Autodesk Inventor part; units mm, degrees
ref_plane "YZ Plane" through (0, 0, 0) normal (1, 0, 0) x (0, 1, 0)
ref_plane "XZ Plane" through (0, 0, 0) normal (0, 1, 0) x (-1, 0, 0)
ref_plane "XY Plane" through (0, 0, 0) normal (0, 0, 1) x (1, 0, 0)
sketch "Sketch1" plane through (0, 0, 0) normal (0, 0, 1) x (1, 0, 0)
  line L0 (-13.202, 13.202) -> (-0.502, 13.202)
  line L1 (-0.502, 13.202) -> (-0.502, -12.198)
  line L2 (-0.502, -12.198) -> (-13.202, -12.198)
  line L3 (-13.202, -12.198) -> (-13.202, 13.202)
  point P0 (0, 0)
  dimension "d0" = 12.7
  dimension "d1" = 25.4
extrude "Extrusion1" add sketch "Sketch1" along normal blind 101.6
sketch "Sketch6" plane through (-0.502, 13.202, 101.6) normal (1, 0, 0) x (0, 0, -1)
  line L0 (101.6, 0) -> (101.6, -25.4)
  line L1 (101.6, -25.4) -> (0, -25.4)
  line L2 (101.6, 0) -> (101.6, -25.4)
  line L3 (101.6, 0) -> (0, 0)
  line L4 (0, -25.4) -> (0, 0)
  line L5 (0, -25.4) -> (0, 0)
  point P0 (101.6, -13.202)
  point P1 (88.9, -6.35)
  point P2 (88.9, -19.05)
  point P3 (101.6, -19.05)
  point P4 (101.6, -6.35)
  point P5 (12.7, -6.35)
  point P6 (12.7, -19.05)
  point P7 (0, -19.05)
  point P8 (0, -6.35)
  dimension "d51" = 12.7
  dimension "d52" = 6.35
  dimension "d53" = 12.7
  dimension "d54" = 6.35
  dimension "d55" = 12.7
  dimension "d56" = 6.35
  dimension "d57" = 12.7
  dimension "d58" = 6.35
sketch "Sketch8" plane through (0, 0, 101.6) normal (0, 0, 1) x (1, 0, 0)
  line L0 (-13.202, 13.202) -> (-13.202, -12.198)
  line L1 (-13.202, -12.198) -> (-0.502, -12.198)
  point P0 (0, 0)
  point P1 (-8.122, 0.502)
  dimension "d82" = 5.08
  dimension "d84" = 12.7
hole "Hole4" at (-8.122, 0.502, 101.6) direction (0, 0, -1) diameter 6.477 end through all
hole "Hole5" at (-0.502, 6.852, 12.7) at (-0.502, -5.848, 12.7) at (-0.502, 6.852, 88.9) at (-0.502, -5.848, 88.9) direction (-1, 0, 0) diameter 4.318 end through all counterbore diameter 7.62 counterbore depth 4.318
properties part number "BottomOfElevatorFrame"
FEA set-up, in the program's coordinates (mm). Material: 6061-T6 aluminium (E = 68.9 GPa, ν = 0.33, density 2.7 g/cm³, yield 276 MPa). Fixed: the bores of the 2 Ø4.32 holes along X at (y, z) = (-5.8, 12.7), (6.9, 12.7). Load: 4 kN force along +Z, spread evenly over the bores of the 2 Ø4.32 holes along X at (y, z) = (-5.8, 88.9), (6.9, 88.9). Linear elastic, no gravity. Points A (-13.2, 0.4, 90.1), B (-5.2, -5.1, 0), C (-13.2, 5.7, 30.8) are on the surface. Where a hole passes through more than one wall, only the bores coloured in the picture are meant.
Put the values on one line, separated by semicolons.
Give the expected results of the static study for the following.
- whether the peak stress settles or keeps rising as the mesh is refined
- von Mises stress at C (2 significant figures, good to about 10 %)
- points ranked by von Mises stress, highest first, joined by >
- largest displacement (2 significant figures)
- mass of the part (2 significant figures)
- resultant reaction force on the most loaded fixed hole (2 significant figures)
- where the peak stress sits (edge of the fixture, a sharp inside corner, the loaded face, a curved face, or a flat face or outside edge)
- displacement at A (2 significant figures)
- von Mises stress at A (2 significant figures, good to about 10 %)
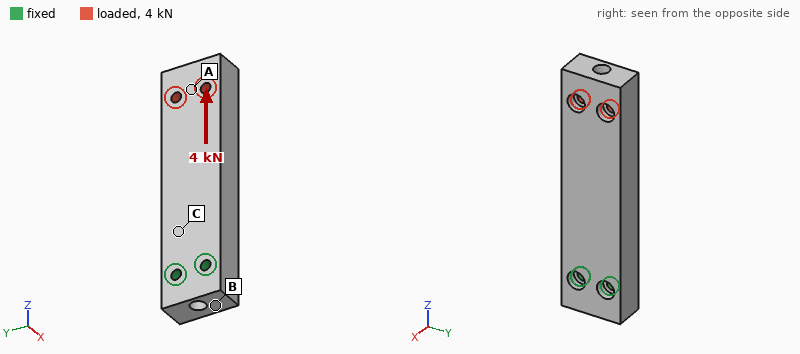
keeps rising; 28 MPa; C > A > B; 0.12 mm; 76 g; 2.0 kN; edge of the fixture; 0.091 mm; 16 MPa
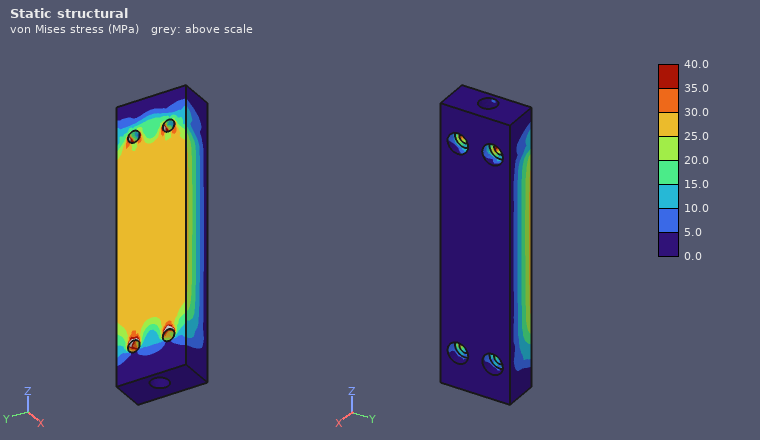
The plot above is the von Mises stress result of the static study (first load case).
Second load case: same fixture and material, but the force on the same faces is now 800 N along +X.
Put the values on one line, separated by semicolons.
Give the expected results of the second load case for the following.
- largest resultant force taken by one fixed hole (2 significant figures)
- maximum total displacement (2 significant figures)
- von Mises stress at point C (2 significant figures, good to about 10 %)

420 N; 0.65 mm; 72 MPa
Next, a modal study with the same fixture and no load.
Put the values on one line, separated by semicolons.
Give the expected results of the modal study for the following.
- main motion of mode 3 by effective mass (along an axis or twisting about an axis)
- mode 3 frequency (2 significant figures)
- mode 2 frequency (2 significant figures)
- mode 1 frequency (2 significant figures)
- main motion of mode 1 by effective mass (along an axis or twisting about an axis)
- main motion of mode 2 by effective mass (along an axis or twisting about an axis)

twisting about Z; 6400 Hz; 2400 Hz; 1200 Hz; along X; along Y
